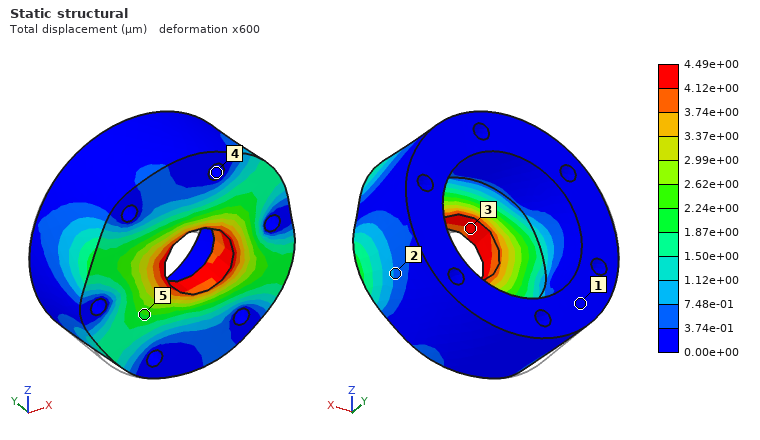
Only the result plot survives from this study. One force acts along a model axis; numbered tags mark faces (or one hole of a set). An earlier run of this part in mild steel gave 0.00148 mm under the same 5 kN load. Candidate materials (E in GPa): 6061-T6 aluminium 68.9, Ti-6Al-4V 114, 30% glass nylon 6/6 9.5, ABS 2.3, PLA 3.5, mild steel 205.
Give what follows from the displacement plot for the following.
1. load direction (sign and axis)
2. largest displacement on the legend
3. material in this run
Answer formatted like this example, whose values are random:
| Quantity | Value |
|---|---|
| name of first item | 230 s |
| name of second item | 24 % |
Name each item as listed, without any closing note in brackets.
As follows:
| Quantity | Value |
|---|---|
| load direction | +X |
| largest displacement on the legend | 4.49e+00 µm |
| material in this run | 6061-T6 aluminium |
